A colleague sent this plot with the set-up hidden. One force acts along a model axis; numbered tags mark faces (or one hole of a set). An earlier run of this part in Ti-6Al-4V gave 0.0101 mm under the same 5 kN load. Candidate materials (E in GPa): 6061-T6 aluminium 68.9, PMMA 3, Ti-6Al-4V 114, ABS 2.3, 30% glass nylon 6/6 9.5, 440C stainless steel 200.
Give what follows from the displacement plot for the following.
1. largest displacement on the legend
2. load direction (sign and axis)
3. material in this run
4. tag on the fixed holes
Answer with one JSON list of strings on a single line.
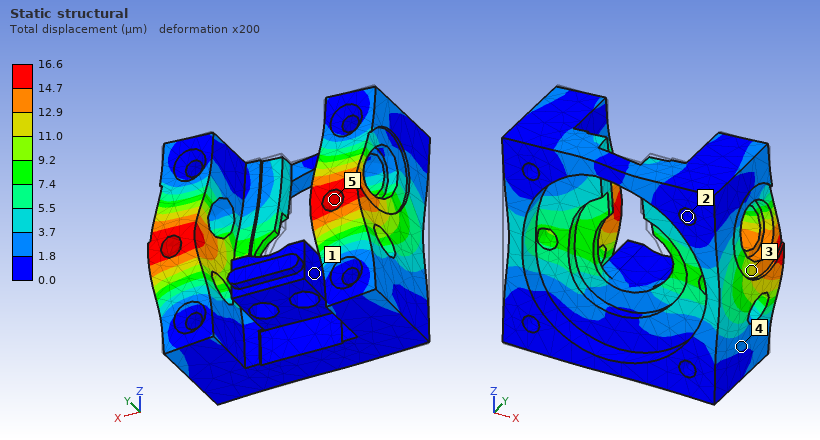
["16.6 µm", "+X", "6061-T6 aluminium", "2"]
